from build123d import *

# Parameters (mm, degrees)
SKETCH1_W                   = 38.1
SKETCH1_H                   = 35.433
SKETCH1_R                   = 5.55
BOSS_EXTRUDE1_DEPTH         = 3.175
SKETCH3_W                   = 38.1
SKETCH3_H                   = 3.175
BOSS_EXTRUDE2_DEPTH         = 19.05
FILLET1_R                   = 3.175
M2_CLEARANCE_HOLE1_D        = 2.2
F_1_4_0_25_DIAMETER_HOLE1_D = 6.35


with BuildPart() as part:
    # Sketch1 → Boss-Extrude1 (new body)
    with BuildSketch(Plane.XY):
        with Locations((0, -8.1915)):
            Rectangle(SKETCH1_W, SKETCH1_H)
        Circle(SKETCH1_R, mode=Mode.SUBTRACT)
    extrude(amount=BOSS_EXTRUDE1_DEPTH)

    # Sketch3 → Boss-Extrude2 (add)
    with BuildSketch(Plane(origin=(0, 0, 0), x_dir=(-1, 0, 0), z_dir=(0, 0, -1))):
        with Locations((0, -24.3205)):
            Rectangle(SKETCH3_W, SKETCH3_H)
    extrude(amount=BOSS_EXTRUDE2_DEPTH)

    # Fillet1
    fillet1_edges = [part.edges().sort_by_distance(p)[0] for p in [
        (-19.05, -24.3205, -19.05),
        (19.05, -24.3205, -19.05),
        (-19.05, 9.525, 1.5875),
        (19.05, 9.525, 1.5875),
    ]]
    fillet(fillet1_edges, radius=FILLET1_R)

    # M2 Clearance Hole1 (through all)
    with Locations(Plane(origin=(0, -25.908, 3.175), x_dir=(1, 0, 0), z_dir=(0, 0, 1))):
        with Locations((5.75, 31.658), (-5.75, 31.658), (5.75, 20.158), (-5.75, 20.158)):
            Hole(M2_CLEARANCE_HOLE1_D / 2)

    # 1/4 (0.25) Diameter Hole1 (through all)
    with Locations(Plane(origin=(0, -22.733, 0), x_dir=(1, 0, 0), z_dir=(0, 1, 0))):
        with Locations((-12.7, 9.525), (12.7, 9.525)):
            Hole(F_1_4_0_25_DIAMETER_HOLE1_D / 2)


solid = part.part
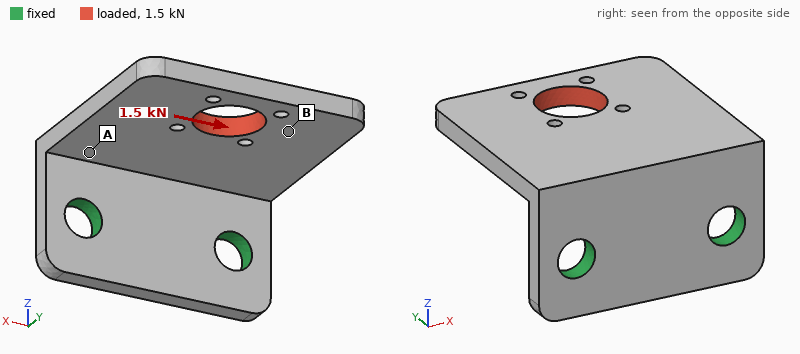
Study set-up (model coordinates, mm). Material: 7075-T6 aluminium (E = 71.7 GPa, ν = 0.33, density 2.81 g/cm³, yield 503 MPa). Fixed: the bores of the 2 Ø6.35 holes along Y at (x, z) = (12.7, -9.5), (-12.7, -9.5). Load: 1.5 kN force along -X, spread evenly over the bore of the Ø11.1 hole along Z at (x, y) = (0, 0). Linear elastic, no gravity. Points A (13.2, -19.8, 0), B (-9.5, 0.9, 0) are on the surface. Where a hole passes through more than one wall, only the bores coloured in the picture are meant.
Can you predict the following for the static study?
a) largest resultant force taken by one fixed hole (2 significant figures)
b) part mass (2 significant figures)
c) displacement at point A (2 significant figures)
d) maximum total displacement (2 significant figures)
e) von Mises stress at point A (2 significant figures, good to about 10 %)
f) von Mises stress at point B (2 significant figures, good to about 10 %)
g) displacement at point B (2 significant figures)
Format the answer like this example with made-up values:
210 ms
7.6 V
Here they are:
1.6 kN
17 g
0.077 mm
0.27 mm
120 MPa
35 MPa
0.19 mm
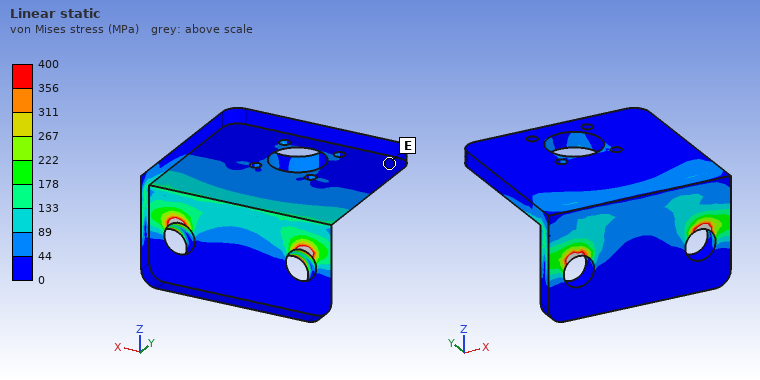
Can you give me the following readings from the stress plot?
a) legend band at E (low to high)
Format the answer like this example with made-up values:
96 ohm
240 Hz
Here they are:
0 to 44 MPa
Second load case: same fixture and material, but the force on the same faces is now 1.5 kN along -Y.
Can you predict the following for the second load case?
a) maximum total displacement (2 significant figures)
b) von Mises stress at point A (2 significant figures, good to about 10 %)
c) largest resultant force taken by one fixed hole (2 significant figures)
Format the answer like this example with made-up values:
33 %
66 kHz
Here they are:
0.31 mm
24 MPa
750 N
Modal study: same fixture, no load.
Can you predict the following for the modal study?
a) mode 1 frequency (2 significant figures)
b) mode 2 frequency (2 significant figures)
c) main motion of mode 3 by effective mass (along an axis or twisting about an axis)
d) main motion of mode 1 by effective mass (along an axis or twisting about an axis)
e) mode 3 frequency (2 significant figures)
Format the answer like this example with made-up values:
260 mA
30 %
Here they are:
1800 Hz
4000 Hz
along X
along Z
6100 Hz
